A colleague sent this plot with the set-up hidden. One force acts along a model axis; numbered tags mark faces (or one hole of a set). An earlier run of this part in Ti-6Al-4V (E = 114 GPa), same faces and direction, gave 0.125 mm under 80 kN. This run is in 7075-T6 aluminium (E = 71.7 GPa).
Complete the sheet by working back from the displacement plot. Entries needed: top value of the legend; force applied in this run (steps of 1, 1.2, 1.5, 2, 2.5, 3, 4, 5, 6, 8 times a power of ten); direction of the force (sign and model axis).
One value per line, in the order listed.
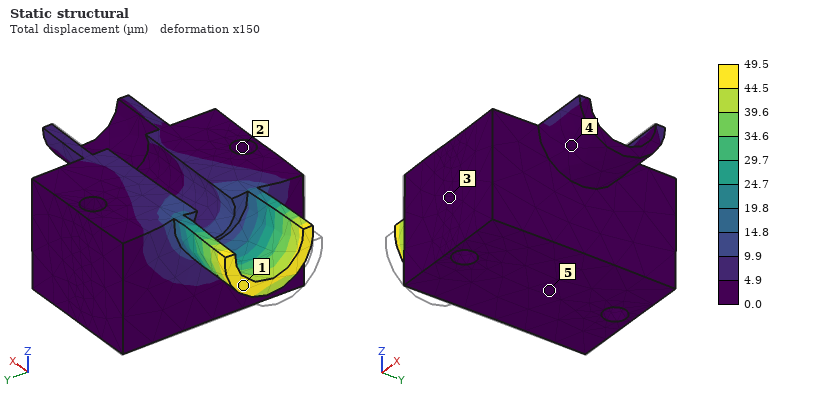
49.5 µm
20 kN
+X
